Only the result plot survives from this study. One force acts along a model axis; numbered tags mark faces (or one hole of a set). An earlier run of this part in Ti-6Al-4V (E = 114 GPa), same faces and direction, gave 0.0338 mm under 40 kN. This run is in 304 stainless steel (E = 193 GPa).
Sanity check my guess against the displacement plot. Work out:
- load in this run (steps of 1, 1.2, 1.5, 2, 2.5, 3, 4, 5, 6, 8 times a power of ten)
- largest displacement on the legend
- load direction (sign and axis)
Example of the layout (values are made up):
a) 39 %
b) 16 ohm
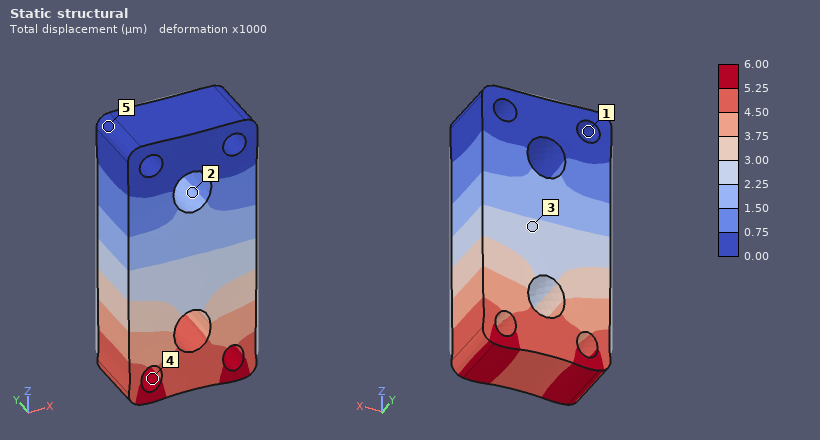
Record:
a) 12 kN
b) 6.00 µm
c) -Z
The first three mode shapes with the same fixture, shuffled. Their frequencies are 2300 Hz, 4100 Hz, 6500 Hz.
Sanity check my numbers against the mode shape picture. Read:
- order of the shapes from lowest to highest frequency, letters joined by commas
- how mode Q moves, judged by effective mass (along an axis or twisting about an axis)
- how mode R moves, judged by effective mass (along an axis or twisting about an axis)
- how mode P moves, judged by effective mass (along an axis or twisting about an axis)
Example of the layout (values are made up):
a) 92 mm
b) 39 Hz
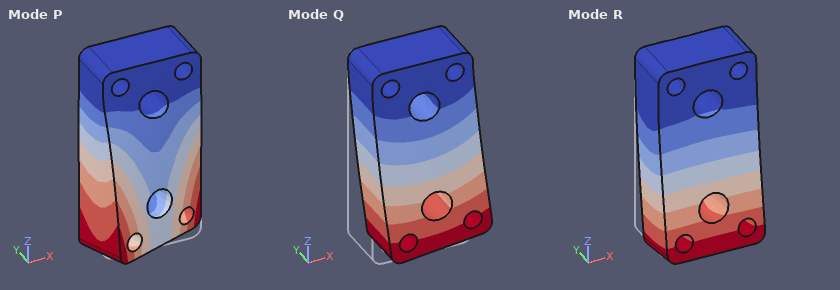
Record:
a) R, Q, P
b) along X
c) along Y
d) twisting about Z
